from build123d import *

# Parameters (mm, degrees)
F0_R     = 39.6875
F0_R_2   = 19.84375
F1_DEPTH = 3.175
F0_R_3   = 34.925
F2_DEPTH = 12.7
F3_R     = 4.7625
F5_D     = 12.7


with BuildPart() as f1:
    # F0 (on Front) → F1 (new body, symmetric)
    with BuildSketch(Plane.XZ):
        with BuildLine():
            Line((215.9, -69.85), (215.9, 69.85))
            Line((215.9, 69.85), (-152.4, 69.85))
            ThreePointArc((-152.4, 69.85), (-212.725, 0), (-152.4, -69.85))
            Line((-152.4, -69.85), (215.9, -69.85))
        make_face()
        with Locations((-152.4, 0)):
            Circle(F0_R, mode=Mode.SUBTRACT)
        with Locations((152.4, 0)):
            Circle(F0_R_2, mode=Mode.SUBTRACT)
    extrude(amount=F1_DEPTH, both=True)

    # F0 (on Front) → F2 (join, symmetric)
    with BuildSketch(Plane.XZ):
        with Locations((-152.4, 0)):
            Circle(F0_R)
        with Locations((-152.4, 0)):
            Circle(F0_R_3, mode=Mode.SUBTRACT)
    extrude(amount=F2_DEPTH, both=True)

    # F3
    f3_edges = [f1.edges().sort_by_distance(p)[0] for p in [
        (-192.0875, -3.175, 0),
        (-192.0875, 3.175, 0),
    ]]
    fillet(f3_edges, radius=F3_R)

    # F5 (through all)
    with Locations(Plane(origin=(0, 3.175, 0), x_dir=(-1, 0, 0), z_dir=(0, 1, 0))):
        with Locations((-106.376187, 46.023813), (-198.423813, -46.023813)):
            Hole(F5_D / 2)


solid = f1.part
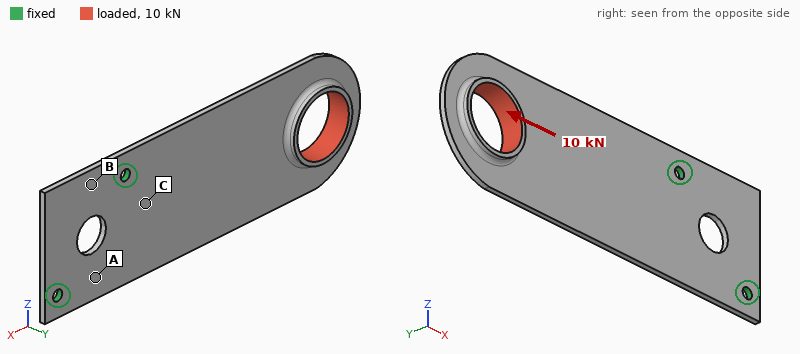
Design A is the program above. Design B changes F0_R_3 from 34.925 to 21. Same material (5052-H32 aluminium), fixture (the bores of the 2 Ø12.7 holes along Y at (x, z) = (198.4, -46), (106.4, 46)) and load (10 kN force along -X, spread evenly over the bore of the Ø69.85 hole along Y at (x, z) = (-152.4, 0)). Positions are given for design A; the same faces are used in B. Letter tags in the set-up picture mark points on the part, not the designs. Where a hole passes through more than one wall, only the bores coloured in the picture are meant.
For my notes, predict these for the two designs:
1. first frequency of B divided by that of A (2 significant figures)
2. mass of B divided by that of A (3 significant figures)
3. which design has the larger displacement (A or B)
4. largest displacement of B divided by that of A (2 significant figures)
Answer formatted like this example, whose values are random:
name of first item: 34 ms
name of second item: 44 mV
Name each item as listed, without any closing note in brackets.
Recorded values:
first frequency of B divided by that of A: 0.80
mass of B divided by that of A: 1.17
which design has the larger displacement: A
largest displacement of B divided by that of A: 0.87
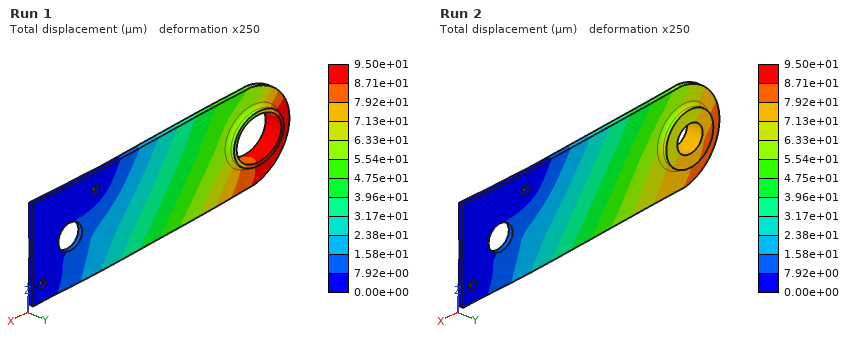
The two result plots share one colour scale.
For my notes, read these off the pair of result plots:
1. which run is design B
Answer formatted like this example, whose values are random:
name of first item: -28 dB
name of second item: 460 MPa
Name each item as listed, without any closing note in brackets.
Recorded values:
which run is design B: Run 2
